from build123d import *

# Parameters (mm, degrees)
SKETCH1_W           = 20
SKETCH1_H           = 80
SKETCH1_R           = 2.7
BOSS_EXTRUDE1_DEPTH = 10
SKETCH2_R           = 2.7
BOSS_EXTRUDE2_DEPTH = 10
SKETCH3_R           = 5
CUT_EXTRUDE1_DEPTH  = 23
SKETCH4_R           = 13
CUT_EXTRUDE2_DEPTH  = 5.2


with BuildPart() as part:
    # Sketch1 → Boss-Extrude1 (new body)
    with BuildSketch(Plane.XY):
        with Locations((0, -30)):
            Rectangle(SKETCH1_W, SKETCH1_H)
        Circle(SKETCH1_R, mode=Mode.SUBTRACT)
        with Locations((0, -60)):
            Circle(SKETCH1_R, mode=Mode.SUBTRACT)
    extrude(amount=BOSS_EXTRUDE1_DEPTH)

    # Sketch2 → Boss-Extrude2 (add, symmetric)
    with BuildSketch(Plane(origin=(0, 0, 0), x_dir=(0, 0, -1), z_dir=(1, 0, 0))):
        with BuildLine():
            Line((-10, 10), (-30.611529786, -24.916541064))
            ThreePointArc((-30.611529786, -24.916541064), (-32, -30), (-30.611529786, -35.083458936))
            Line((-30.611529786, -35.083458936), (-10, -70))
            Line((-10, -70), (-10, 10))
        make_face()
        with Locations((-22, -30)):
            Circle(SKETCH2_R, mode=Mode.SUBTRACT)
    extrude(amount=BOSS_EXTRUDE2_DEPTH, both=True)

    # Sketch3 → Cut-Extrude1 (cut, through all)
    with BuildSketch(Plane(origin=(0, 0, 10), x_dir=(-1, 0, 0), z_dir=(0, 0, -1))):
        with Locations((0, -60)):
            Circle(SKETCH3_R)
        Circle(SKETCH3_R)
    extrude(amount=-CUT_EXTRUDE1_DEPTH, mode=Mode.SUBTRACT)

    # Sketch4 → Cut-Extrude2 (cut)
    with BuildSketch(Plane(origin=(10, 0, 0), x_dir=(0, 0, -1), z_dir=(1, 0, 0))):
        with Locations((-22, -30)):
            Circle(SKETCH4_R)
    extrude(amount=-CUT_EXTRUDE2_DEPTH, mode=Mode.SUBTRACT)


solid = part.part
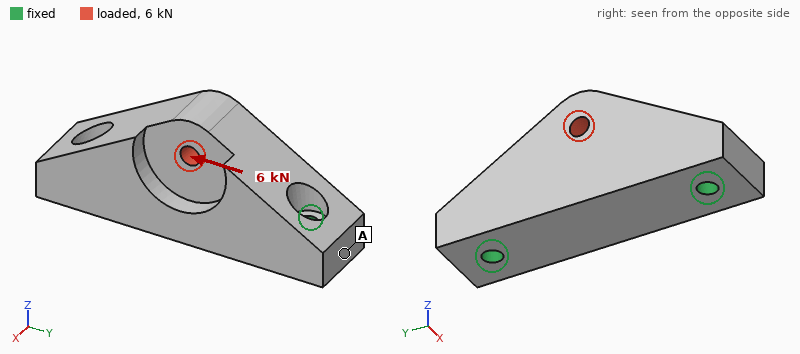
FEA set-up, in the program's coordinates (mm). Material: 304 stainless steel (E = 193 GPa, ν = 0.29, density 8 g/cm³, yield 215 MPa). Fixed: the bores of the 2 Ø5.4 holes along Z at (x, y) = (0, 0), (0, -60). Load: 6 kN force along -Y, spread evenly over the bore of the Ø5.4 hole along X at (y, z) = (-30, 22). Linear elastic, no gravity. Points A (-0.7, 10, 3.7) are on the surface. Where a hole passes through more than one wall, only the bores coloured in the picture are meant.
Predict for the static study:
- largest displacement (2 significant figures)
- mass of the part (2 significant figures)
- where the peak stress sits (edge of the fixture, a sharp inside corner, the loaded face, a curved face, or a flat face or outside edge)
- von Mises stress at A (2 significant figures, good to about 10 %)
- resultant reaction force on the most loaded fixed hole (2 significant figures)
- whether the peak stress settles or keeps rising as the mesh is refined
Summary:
3.8 µm
250 g
a sharp inside corner
9.0 MPa
3.4 kN
keeps rising
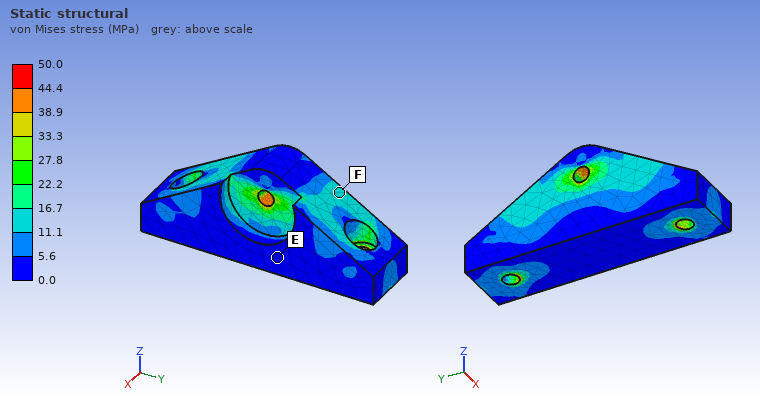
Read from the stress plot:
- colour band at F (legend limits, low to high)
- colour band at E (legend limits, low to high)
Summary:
11.1 to 16.7 MPa
0.0 to 5.6 MPa
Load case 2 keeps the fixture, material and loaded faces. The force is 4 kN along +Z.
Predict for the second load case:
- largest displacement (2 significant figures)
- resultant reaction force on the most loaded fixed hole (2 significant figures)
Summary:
6.1 µm
2.4 kN
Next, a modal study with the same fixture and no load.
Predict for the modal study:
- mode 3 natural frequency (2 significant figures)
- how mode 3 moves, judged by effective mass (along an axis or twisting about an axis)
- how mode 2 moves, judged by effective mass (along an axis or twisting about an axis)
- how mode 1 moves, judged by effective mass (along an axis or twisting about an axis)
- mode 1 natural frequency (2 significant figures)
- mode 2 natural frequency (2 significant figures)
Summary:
16 kHz
along X
along Z
along X
8400 Hz
15 kHz
